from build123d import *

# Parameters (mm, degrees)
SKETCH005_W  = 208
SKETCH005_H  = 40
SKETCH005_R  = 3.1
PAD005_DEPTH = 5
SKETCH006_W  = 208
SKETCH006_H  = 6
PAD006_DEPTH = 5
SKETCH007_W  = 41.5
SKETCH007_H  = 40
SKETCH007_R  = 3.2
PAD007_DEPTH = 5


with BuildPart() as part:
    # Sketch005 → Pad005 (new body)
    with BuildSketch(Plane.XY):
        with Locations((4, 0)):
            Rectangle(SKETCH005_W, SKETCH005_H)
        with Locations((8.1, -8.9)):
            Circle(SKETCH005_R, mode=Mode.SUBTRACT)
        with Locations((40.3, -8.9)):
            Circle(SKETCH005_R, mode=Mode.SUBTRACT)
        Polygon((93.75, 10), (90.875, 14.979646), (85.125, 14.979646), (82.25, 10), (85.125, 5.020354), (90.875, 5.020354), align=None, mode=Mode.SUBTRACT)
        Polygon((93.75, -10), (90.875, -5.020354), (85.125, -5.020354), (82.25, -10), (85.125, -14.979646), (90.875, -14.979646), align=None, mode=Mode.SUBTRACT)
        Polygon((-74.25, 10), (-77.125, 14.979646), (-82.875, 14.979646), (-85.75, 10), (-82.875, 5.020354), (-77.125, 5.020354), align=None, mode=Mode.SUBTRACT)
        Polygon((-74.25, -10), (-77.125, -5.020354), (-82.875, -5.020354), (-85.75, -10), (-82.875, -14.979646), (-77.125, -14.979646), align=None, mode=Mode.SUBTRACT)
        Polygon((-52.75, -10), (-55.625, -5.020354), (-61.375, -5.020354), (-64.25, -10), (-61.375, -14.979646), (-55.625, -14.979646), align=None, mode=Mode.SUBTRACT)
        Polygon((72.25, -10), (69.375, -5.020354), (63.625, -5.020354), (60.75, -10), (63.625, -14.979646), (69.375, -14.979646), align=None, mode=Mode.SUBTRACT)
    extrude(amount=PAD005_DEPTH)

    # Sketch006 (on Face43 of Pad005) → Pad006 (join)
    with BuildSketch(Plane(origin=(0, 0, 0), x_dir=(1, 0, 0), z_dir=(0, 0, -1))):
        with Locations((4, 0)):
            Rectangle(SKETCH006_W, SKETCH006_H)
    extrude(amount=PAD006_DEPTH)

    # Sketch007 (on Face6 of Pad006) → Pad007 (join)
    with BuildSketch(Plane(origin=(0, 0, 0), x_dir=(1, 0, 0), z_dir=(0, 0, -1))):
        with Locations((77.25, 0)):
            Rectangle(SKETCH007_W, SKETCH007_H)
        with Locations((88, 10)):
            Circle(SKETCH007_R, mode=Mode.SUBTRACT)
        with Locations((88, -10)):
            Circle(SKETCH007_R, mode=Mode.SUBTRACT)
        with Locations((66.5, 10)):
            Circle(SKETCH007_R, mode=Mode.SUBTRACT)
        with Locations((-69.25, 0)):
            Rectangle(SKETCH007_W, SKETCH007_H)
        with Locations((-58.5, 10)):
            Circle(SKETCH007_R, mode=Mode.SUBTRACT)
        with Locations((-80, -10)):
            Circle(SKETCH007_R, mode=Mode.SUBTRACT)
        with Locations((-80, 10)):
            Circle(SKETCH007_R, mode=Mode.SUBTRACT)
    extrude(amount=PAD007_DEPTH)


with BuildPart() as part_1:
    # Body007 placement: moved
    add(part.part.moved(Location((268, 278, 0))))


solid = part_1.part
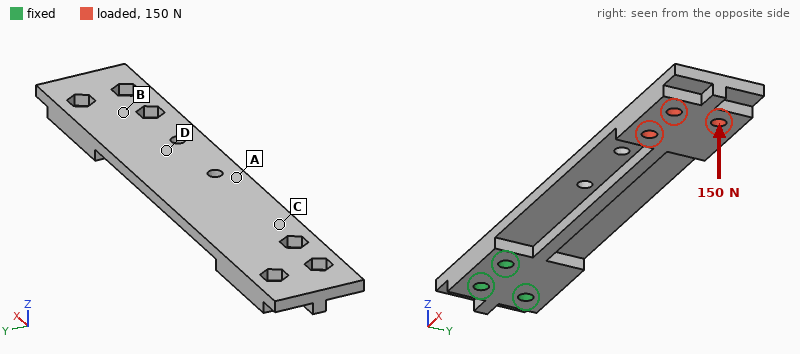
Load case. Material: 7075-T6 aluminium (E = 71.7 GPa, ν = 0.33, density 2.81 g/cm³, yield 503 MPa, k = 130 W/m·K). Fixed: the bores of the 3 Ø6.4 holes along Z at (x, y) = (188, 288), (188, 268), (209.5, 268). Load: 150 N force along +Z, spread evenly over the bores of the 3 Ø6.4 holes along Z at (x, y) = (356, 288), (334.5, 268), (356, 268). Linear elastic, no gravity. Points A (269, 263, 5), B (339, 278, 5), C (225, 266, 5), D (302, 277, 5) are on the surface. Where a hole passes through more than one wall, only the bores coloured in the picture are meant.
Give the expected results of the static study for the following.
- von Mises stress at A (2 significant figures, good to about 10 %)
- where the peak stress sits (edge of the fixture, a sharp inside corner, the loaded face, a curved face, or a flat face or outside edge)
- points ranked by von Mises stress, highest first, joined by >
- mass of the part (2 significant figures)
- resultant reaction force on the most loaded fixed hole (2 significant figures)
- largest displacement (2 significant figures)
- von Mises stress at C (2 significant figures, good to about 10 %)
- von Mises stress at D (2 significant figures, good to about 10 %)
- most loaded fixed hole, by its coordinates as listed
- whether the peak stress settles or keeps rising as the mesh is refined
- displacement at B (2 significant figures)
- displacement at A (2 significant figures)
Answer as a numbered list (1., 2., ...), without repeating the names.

1. 35 MPa
2. edge of the fixture
3. C > A > D > B
4. 160 g
5. 960 N
6. 2.1 mm
7. 50 MPa
8. 20 MPa
9. (209.5, 268)
10. keeps rising
11. 1.5 mm
12. 0.38 mm
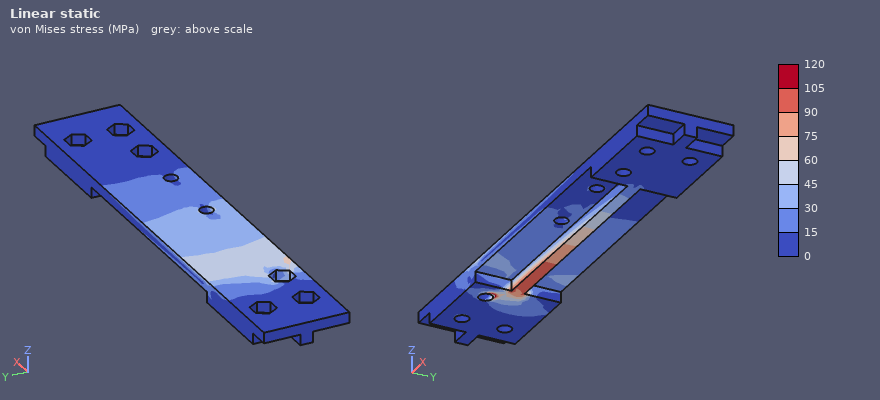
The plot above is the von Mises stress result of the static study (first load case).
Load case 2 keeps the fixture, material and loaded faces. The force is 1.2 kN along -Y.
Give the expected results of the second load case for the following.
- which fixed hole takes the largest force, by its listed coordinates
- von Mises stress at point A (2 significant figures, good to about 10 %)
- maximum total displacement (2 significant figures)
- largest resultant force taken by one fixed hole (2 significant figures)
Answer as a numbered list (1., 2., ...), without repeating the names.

1. (209.5, 268)
2. 64 MPa
3. 0.99 mm
4. 5.3 kN
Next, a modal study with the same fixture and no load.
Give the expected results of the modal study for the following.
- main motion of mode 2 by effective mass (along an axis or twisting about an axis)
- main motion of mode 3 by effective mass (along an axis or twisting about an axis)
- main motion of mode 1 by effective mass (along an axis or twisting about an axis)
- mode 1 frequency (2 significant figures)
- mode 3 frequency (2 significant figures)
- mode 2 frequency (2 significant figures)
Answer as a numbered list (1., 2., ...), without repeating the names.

1. along Y
2. twisting about X
3. along Z
4. 200 Hz
5. 1200 Hz
6. 840 Hz
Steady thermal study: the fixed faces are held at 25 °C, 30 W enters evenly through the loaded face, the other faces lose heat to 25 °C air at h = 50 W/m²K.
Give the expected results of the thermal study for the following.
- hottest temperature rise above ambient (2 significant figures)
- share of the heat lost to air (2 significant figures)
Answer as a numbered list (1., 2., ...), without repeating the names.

1. 50 K
2. 78 %
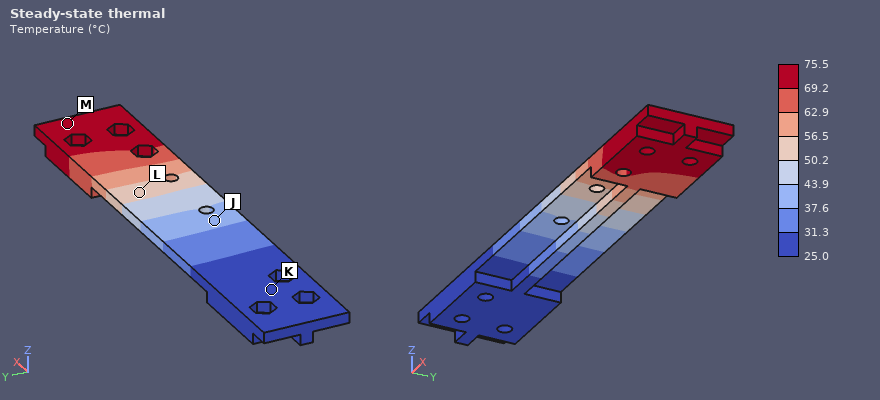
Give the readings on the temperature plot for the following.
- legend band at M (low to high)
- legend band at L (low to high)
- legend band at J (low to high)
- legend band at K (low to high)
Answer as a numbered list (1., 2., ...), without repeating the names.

1. 69.2 to 75.5 °C
2. 50.2 to 56.5 °C
3. 37.6 to 43.9 °C
4. 25.0 to 31.3 °C
